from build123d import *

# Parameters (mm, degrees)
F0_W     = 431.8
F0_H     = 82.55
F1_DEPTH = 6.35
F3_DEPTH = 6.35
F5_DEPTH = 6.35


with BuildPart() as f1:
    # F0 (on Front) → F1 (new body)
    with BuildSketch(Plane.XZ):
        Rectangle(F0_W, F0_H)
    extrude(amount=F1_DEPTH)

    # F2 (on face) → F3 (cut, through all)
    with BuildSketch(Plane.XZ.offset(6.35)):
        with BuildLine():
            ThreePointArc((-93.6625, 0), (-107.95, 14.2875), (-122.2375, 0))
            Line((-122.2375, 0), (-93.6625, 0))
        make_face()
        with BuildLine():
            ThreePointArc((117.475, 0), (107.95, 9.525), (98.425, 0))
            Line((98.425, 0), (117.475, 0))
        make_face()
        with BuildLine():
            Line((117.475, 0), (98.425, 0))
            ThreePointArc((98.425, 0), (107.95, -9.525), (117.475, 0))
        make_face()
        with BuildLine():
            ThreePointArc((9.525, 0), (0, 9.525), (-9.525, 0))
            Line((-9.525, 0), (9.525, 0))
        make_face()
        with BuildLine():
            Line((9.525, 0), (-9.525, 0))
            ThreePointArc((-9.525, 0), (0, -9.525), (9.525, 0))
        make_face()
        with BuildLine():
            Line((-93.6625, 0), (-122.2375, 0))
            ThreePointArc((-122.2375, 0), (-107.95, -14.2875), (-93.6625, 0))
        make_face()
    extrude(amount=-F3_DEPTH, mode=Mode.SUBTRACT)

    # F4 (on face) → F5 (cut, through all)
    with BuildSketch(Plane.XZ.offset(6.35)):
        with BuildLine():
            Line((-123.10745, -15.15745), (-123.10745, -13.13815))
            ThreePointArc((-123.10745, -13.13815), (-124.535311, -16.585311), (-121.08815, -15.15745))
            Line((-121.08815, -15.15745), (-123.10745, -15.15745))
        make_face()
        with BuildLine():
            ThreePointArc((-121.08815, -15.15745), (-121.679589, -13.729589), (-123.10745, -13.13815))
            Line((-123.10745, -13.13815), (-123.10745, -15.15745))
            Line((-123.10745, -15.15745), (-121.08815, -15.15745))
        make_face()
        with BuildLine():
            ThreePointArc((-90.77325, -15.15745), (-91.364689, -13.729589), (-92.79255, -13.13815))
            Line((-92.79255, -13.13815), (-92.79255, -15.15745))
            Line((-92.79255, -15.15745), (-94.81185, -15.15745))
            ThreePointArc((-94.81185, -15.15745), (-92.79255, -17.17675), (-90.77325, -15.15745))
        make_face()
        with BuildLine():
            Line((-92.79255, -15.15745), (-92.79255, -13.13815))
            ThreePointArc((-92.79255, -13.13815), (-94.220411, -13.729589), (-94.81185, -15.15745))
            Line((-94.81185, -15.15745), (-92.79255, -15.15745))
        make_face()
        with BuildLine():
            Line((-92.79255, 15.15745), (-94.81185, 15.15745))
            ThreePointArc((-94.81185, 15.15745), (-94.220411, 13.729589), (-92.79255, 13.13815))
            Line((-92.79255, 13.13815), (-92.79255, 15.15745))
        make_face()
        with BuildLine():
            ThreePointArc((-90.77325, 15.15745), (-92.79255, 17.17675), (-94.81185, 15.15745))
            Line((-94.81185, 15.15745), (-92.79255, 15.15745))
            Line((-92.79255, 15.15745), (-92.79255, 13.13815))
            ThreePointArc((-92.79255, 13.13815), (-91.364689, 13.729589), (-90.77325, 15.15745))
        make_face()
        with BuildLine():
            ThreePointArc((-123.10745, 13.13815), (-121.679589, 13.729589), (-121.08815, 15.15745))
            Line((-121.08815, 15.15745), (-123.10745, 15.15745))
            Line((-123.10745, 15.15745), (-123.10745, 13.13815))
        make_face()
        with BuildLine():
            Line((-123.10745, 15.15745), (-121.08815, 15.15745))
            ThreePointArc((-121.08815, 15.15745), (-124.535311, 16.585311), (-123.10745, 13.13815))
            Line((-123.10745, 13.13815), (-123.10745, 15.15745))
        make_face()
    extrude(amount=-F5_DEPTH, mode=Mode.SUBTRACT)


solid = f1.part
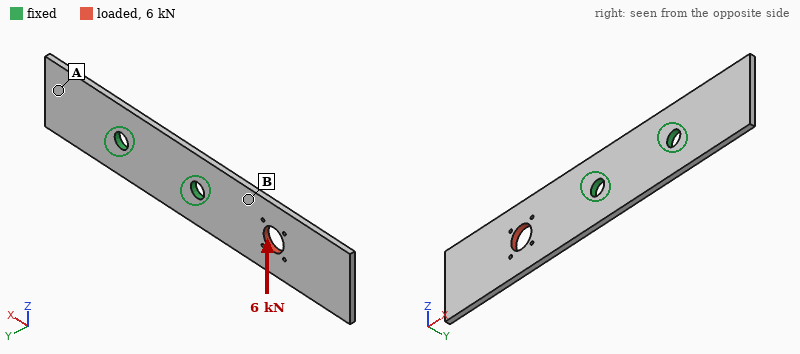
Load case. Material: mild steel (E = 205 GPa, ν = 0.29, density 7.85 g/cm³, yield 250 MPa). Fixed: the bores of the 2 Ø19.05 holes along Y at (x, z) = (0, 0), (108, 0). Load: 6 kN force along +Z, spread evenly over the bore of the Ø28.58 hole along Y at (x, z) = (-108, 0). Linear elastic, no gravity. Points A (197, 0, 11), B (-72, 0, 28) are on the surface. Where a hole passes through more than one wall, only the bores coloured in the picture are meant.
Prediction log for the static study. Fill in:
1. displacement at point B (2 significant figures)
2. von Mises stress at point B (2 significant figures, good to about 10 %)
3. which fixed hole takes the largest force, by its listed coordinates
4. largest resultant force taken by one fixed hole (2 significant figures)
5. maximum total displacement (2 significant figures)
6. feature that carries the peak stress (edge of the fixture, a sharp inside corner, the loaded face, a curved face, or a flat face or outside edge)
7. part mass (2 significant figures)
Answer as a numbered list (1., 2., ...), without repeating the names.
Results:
1. 0.063 mm
2. 23 MPa
3. (0, 0)
4. 9.9 kN
5. 0.21 mm
6. edge of the fixture
7. 1.7 kg
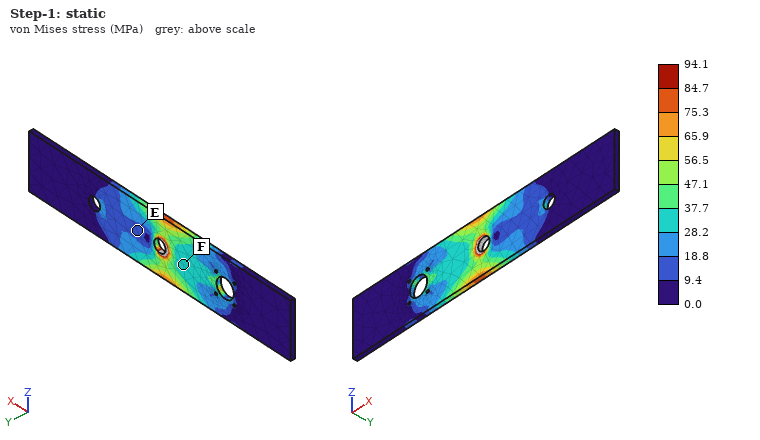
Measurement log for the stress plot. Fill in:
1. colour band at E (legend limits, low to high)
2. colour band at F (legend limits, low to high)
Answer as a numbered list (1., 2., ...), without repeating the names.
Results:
1. 9.4 to 18.8 MPa
2. 28.2 to 37.7 MPa
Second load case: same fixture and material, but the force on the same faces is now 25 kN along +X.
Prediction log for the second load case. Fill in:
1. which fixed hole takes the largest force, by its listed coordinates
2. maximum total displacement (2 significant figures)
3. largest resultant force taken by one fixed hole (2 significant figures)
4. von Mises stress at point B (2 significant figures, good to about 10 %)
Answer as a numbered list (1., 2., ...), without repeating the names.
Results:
1. (0, 0)
2. 37 µm
3. 22 kN
4. 49 MPa
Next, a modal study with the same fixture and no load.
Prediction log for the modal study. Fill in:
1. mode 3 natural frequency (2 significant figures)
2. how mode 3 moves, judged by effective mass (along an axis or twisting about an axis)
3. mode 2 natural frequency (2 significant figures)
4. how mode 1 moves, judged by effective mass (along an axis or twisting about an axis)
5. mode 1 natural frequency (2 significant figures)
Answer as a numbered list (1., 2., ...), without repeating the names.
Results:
1. 560 Hz
2. twisting about X
3. 490 Hz
4. along Y
5. 120 Hz
